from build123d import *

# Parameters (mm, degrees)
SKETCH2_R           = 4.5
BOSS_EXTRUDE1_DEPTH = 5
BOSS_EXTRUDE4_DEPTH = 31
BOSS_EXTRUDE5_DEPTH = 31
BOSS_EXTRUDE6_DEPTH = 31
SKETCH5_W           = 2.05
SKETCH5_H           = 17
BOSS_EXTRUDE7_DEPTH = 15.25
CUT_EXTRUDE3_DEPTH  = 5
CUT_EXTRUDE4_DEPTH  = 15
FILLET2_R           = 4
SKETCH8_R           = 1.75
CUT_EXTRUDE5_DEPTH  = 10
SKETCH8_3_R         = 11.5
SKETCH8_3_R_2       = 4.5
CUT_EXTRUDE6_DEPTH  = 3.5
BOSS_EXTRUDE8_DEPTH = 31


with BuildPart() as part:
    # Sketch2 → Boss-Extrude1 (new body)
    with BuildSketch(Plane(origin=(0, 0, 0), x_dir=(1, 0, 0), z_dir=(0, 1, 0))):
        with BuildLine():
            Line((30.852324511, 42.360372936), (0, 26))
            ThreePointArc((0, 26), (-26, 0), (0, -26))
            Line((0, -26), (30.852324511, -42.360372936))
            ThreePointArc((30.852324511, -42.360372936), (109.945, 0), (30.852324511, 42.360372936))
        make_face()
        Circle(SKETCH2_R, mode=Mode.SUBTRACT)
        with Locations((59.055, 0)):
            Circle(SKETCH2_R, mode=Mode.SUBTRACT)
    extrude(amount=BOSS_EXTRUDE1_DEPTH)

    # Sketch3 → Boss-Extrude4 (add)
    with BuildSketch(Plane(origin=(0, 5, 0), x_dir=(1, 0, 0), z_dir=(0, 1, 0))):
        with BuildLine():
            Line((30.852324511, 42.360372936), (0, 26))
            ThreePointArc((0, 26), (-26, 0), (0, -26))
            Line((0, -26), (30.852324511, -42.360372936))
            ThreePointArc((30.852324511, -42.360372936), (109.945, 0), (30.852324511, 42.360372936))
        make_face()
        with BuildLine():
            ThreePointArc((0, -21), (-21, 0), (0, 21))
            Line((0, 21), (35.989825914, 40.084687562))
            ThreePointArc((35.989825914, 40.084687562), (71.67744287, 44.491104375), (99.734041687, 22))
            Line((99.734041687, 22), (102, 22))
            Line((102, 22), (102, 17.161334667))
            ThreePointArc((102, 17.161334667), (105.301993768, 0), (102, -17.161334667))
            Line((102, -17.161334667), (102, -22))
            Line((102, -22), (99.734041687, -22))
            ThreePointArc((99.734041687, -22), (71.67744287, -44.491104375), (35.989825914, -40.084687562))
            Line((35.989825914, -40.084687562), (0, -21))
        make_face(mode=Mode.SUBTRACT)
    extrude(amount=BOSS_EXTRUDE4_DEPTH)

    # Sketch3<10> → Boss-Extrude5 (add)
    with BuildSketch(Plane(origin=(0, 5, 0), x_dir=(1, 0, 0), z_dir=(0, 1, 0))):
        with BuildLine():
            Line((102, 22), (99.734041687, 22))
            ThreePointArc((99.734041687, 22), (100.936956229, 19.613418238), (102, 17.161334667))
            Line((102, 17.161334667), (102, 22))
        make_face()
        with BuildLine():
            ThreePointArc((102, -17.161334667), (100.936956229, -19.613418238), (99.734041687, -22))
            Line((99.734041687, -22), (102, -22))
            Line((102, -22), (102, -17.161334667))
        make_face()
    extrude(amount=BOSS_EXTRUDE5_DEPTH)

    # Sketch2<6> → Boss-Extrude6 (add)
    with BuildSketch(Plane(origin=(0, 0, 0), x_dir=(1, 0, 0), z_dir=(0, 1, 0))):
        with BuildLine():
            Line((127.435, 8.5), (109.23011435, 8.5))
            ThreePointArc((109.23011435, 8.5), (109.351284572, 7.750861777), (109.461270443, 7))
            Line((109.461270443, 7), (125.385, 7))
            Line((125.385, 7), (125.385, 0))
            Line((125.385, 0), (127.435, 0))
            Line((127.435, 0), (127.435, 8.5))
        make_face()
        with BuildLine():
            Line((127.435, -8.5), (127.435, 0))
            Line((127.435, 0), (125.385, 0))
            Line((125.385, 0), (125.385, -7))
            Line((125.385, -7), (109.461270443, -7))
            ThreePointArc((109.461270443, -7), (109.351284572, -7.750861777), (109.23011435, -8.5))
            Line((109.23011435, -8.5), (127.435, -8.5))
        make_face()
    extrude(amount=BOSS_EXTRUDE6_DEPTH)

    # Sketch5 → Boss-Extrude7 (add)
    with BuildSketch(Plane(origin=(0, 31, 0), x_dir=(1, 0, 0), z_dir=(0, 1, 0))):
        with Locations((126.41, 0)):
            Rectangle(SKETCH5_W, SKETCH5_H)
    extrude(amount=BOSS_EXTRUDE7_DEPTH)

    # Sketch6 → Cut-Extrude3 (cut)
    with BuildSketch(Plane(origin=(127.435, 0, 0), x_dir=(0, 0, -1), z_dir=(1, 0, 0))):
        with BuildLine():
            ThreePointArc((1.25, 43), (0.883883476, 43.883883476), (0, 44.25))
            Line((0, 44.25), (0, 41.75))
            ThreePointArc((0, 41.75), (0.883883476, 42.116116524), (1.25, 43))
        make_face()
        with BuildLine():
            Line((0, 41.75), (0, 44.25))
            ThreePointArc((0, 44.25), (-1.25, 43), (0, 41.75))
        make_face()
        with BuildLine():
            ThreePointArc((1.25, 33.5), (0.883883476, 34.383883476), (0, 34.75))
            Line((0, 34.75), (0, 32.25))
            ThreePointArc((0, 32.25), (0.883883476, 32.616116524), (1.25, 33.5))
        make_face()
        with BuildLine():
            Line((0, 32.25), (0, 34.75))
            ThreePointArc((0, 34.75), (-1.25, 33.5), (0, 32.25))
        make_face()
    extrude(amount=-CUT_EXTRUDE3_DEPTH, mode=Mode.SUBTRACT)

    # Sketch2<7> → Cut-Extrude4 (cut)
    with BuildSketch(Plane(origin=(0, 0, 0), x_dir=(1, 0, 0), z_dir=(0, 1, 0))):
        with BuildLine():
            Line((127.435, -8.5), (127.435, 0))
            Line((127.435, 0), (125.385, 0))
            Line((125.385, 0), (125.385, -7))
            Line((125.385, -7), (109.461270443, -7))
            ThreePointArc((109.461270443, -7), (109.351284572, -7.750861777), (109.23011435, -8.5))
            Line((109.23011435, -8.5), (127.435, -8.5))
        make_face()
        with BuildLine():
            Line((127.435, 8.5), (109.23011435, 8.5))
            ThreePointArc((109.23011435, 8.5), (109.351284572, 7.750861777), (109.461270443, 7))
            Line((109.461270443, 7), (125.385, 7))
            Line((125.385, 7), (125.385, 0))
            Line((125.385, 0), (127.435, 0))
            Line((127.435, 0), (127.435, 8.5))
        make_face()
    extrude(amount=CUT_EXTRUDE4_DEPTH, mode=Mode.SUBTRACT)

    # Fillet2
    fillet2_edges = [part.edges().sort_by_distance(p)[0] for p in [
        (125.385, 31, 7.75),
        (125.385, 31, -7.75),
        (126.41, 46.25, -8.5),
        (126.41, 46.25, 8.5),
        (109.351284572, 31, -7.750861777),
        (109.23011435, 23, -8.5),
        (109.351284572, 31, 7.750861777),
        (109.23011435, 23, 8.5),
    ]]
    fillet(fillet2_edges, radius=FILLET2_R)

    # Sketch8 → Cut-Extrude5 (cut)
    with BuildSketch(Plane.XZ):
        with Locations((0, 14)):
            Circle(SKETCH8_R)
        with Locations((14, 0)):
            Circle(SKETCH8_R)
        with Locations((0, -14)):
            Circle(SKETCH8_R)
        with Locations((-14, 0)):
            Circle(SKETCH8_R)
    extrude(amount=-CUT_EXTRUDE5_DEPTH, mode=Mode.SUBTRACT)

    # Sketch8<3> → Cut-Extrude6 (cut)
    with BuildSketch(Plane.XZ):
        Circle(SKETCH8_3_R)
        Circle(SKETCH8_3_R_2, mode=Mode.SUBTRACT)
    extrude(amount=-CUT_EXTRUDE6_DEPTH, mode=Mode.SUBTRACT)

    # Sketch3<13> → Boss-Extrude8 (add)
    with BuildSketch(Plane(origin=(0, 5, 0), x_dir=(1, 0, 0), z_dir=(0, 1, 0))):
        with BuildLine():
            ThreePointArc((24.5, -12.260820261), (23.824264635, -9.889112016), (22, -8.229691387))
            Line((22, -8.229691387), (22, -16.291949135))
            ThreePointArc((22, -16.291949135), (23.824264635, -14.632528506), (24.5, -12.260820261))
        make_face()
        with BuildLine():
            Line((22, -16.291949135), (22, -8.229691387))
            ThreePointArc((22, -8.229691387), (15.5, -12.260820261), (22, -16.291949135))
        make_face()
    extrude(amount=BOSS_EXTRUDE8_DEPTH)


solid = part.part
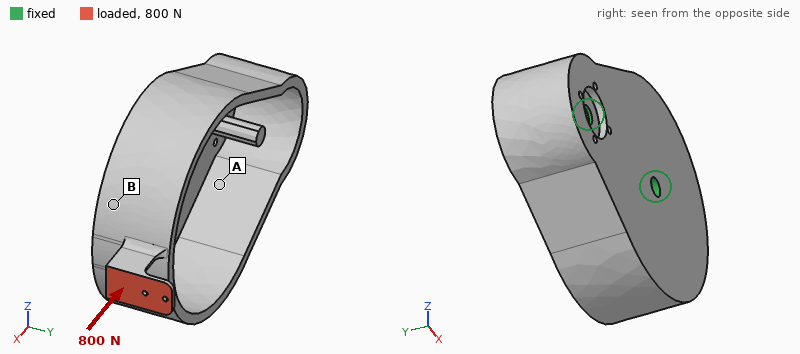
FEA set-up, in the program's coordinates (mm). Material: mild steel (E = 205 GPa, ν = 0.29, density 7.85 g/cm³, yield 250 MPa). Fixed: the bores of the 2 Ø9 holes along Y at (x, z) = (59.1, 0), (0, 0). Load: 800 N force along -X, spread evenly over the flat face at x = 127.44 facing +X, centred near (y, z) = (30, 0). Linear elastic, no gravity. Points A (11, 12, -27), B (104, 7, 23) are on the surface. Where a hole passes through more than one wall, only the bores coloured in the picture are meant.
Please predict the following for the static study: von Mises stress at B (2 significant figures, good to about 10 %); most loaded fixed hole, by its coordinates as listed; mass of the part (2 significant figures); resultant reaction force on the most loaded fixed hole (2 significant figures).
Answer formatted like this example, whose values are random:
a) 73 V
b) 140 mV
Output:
a) 25 MPa
b) (59.1, 0)
c) 810 g
d) 640 N
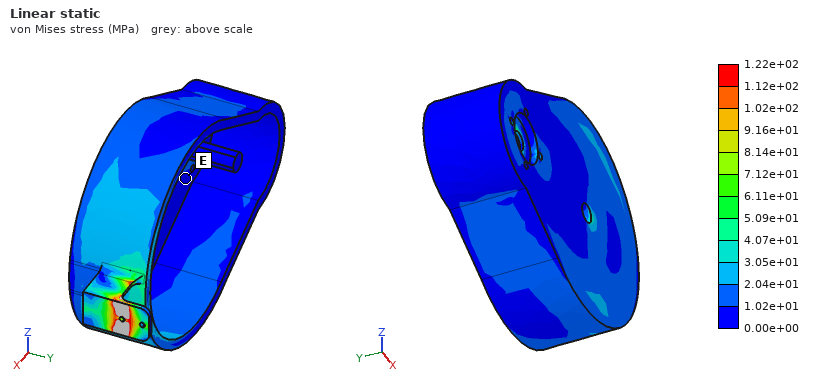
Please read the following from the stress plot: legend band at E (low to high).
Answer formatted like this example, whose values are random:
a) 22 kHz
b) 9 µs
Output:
a) 0.00e+00 to 1.02e+01 MPa
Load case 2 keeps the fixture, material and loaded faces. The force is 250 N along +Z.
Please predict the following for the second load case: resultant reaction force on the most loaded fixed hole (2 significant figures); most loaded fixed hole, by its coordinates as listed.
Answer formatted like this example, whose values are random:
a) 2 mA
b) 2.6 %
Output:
a) 480 N
b) (59.1, 0)
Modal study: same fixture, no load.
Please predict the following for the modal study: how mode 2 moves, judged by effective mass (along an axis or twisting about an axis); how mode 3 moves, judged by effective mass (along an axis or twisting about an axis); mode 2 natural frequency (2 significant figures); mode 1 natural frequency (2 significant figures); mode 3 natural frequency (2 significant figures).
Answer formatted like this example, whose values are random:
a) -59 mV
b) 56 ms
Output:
a) along Y
b) along Y
c) 1200 Hz
d) 760 Hz
e) 1600 Hz
